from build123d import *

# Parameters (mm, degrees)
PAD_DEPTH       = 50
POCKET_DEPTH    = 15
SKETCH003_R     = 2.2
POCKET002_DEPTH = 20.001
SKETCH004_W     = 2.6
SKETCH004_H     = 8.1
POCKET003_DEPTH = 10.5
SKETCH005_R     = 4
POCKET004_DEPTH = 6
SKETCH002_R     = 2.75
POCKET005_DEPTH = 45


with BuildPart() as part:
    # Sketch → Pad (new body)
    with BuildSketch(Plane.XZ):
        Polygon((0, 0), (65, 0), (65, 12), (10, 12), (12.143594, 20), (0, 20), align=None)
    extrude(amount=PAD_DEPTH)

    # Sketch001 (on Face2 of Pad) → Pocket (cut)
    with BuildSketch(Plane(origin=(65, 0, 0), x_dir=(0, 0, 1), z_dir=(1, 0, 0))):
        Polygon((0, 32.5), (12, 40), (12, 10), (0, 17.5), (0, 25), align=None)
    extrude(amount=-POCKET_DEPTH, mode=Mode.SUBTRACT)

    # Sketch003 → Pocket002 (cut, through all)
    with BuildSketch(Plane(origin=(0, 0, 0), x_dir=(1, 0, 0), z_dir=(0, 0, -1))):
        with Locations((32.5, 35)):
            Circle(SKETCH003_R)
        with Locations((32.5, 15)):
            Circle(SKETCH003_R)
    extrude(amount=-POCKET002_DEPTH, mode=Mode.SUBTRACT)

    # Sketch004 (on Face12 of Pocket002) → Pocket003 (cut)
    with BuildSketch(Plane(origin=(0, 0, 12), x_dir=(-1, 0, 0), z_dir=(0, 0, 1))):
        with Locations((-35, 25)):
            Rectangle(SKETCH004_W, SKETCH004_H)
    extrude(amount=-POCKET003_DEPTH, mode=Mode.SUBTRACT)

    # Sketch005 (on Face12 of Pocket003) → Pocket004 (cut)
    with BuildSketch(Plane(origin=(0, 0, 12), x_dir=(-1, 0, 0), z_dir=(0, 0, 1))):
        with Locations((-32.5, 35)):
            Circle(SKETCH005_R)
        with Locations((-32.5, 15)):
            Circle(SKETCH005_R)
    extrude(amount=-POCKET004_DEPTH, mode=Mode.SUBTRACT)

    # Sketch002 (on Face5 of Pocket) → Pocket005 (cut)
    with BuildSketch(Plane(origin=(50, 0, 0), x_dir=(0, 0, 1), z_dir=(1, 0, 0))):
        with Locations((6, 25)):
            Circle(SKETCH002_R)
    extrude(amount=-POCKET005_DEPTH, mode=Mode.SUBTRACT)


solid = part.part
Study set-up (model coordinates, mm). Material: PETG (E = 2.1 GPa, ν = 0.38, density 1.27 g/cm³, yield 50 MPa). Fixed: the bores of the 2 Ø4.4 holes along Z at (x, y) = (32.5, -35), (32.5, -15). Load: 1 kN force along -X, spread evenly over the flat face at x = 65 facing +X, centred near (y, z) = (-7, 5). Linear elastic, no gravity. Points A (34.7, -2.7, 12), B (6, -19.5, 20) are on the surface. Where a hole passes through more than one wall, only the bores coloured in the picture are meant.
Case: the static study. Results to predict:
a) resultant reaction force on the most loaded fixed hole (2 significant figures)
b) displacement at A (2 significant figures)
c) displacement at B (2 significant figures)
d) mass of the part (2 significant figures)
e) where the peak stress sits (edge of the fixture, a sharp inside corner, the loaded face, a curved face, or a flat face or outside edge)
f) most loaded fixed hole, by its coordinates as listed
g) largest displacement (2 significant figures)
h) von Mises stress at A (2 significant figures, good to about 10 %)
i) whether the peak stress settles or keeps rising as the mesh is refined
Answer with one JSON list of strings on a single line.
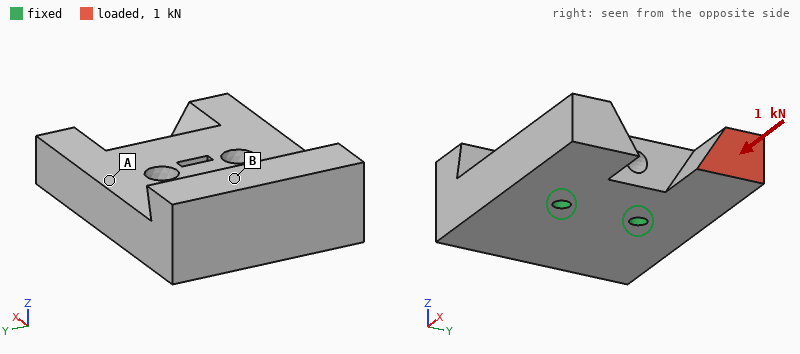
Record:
["1.3 kN", "0.15 mm", "0.17 mm", "47 g", "edge of the fixture", "(32.5, -15)", "0.36 mm", "4.6 MPa", "keeps rising"]
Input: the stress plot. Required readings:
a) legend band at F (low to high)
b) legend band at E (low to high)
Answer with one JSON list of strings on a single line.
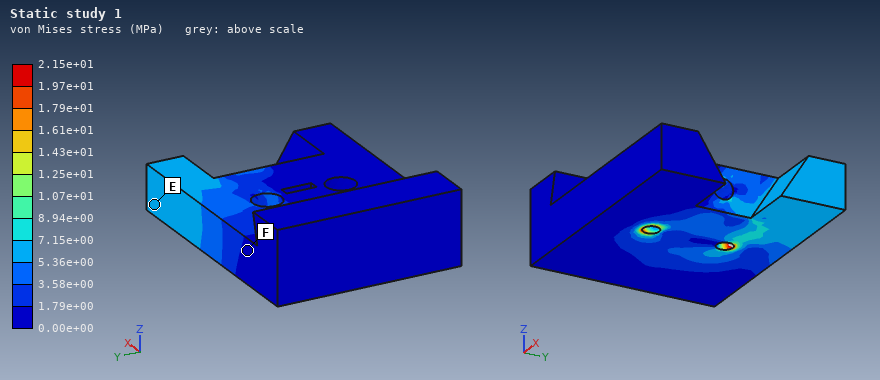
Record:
["0.00e+00 to 1.79e+00 MPa", "5.36e+00 to 7.15e+00 MPa"]
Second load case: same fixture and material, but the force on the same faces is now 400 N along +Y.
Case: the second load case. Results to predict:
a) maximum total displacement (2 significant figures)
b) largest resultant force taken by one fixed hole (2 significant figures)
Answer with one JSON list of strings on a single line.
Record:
["0.54 mm", "610 N"]
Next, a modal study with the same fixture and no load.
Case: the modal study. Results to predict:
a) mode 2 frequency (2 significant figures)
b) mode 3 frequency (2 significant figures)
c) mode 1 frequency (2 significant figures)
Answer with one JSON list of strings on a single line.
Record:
["1900 Hz", "2000 Hz", "810 Hz"]
